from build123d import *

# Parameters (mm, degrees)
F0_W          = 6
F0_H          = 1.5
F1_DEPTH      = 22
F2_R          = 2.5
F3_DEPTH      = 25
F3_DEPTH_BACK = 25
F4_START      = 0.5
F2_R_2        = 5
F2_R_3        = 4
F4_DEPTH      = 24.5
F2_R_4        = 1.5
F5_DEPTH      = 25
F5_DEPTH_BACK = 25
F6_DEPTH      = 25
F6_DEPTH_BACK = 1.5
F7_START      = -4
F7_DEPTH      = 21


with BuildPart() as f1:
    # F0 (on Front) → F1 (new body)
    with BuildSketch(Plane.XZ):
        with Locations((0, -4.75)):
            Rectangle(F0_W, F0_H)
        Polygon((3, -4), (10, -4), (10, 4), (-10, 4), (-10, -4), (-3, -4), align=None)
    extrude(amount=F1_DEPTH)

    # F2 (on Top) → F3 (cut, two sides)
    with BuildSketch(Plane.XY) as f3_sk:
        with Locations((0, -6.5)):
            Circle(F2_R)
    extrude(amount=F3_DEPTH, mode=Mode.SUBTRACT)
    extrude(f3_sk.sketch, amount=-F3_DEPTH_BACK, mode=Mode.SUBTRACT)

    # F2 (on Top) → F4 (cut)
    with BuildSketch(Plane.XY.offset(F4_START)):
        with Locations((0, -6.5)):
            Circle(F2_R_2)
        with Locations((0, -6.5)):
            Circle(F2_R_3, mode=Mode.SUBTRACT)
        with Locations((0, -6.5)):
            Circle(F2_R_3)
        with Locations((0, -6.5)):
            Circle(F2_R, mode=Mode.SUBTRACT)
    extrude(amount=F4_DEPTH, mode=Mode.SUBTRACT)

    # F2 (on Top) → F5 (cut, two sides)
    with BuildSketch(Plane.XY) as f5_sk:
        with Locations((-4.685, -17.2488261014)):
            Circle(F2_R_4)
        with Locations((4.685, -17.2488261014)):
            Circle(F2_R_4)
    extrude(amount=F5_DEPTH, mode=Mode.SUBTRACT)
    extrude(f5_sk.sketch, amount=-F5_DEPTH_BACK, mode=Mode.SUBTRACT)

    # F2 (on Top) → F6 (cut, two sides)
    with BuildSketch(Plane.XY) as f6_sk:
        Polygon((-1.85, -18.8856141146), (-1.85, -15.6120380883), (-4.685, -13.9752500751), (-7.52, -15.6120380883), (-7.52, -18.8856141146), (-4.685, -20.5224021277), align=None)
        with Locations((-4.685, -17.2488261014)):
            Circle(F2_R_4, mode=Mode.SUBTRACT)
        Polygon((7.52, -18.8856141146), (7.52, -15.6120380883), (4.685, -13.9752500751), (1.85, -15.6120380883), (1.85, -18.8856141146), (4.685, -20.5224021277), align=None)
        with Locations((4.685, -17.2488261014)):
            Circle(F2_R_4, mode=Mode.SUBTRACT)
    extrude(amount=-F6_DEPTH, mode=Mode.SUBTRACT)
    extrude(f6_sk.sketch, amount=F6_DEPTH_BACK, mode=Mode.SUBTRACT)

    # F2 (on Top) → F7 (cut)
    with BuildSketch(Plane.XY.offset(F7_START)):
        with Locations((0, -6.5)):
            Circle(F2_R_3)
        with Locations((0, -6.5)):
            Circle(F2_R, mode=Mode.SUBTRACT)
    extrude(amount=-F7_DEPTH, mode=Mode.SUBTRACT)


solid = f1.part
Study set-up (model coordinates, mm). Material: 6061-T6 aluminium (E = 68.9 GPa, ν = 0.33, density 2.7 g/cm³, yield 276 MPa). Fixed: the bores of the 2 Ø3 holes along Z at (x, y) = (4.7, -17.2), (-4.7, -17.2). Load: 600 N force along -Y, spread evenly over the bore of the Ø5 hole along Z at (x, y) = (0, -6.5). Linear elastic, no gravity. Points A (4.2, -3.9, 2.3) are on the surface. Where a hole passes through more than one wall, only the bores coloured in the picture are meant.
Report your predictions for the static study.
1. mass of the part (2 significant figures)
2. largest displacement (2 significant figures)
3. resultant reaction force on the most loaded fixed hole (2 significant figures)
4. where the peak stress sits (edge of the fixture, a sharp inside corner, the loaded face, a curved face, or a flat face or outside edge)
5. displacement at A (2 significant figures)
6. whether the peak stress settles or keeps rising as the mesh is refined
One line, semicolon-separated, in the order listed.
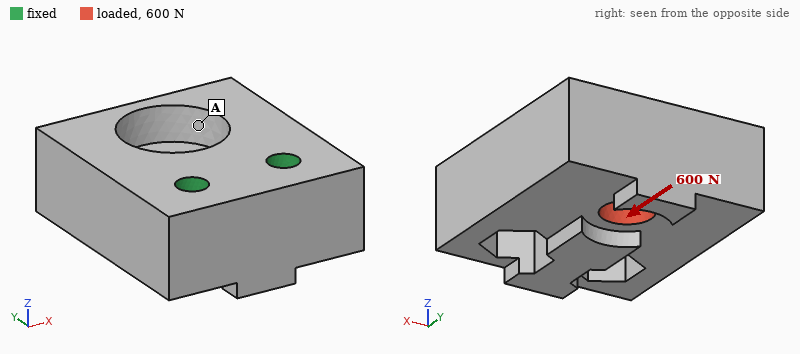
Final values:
7.9 g; 26 µm; 300 N; edge of the fixture; 17 µm; keeps rising
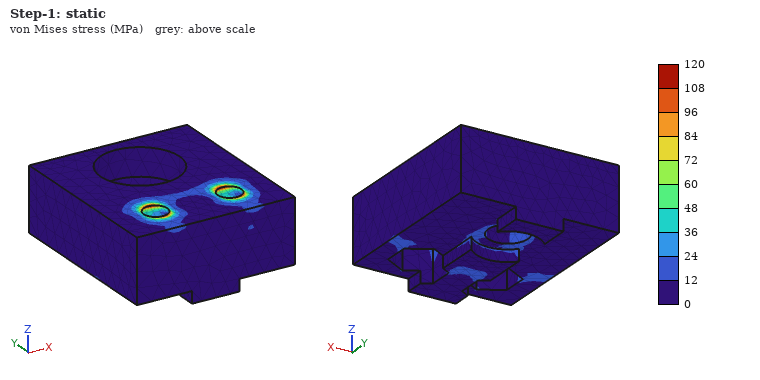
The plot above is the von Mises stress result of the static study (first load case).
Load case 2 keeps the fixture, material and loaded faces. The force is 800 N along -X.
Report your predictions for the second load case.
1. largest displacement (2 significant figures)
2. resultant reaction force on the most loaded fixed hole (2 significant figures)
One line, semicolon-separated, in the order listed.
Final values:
17 µm; 880 N
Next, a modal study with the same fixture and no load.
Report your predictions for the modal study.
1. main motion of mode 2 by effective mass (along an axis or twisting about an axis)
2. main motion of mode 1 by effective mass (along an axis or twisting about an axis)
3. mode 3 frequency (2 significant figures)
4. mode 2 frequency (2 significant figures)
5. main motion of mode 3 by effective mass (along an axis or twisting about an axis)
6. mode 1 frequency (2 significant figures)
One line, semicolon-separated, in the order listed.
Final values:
along X; along Z; 21 kHz; 17 kHz; along X; 8200 Hz
